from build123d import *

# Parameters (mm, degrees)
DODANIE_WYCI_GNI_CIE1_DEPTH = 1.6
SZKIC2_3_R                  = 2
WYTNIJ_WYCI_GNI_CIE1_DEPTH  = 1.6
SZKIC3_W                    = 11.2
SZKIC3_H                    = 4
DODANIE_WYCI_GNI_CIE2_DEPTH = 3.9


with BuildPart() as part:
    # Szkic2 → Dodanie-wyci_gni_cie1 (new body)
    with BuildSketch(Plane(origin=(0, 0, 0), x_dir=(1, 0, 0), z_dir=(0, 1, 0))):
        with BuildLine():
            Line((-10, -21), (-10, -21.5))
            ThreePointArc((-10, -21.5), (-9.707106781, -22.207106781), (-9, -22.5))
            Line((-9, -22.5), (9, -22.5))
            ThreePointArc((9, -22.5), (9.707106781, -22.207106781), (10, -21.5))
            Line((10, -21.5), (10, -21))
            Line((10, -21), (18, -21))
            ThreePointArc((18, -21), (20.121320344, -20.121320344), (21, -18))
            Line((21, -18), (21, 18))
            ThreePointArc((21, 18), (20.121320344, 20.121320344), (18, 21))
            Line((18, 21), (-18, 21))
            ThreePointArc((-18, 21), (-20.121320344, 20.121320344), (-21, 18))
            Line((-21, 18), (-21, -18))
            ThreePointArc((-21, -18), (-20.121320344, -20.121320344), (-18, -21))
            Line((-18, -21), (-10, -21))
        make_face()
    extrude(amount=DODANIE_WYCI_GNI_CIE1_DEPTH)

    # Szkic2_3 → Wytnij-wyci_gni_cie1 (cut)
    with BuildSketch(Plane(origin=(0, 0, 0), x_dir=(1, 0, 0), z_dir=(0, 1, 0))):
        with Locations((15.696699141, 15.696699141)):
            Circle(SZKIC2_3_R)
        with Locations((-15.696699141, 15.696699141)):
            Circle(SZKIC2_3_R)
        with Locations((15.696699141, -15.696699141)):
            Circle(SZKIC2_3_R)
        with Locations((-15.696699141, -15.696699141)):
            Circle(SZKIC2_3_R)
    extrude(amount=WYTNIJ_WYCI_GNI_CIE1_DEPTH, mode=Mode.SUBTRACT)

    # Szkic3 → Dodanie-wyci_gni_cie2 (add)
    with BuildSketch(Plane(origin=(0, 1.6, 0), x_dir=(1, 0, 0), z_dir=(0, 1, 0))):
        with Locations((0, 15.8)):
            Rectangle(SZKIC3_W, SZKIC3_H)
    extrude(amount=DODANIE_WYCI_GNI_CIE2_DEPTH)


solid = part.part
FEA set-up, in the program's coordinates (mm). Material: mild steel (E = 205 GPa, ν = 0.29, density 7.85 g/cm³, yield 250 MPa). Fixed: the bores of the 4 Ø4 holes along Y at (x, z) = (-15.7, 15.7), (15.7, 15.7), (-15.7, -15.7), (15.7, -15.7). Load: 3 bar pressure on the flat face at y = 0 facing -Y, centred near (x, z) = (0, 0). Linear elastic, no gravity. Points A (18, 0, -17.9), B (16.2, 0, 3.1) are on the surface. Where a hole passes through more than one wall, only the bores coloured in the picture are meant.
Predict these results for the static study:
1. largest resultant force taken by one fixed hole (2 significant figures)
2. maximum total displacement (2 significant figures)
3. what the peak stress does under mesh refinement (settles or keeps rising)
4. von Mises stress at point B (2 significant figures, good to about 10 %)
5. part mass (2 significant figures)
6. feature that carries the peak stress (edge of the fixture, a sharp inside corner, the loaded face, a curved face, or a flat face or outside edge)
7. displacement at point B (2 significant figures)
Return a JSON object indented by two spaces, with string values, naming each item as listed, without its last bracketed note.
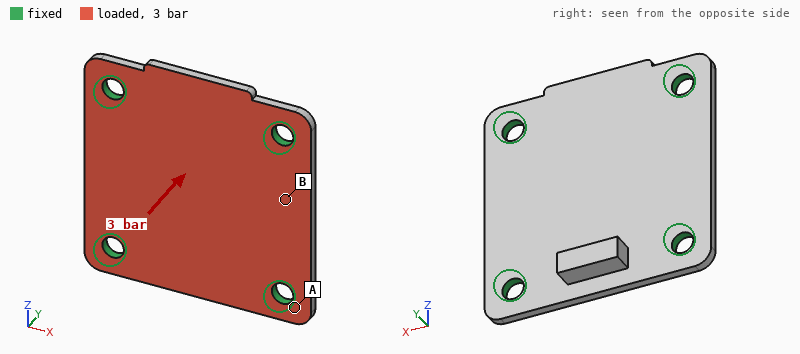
{
  "largest resultant force taken by one fixed hole": "130 N",
  "maximum total displacement": "19 µm",
  "what the peak stress does under mesh refinement": "keeps rising",
  "von Mises stress at point B": "26 MPa",
  "part mass": "23 g",
  "feature that carries the peak stress": "edge of the fixture",
  "displacement at point B": "9.2 µm"
}
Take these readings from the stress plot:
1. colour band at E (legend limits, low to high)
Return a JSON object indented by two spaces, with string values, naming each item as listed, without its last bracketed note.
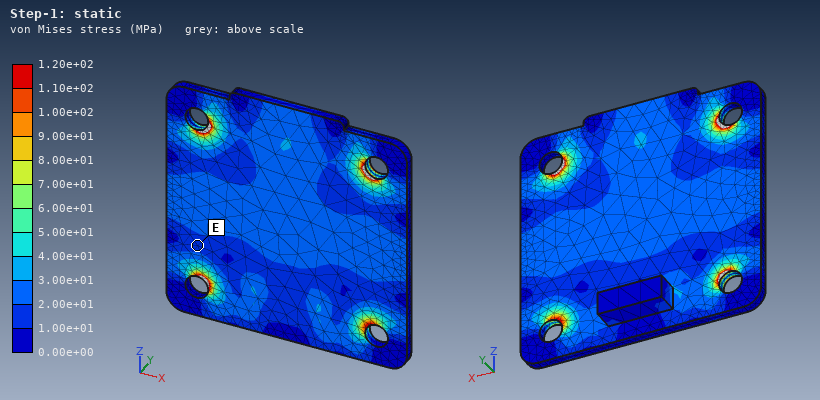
{
  "colour band at E": "1.00e+01 to 2.00e+01 MPa"
}
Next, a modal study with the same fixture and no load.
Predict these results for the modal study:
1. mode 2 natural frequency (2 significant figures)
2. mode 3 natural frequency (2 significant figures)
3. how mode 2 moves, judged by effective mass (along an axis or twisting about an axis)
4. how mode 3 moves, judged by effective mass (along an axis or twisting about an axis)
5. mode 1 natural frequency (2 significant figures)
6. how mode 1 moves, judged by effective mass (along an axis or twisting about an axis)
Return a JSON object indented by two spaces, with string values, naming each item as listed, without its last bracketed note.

{
  "mode 2 natural frequency": "10 kHz",
  "mode 3 natural frequency": "11 kHz",
  "how mode 2 moves, judged by effective mass": "twisting about X",
  "how mode 3 moves, judged by effective mass": "twisting about Z",
  "mode 1 natural frequency": "6900 Hz",
  "how mode 1 moves, judged by effective mass": "along Y"
}
